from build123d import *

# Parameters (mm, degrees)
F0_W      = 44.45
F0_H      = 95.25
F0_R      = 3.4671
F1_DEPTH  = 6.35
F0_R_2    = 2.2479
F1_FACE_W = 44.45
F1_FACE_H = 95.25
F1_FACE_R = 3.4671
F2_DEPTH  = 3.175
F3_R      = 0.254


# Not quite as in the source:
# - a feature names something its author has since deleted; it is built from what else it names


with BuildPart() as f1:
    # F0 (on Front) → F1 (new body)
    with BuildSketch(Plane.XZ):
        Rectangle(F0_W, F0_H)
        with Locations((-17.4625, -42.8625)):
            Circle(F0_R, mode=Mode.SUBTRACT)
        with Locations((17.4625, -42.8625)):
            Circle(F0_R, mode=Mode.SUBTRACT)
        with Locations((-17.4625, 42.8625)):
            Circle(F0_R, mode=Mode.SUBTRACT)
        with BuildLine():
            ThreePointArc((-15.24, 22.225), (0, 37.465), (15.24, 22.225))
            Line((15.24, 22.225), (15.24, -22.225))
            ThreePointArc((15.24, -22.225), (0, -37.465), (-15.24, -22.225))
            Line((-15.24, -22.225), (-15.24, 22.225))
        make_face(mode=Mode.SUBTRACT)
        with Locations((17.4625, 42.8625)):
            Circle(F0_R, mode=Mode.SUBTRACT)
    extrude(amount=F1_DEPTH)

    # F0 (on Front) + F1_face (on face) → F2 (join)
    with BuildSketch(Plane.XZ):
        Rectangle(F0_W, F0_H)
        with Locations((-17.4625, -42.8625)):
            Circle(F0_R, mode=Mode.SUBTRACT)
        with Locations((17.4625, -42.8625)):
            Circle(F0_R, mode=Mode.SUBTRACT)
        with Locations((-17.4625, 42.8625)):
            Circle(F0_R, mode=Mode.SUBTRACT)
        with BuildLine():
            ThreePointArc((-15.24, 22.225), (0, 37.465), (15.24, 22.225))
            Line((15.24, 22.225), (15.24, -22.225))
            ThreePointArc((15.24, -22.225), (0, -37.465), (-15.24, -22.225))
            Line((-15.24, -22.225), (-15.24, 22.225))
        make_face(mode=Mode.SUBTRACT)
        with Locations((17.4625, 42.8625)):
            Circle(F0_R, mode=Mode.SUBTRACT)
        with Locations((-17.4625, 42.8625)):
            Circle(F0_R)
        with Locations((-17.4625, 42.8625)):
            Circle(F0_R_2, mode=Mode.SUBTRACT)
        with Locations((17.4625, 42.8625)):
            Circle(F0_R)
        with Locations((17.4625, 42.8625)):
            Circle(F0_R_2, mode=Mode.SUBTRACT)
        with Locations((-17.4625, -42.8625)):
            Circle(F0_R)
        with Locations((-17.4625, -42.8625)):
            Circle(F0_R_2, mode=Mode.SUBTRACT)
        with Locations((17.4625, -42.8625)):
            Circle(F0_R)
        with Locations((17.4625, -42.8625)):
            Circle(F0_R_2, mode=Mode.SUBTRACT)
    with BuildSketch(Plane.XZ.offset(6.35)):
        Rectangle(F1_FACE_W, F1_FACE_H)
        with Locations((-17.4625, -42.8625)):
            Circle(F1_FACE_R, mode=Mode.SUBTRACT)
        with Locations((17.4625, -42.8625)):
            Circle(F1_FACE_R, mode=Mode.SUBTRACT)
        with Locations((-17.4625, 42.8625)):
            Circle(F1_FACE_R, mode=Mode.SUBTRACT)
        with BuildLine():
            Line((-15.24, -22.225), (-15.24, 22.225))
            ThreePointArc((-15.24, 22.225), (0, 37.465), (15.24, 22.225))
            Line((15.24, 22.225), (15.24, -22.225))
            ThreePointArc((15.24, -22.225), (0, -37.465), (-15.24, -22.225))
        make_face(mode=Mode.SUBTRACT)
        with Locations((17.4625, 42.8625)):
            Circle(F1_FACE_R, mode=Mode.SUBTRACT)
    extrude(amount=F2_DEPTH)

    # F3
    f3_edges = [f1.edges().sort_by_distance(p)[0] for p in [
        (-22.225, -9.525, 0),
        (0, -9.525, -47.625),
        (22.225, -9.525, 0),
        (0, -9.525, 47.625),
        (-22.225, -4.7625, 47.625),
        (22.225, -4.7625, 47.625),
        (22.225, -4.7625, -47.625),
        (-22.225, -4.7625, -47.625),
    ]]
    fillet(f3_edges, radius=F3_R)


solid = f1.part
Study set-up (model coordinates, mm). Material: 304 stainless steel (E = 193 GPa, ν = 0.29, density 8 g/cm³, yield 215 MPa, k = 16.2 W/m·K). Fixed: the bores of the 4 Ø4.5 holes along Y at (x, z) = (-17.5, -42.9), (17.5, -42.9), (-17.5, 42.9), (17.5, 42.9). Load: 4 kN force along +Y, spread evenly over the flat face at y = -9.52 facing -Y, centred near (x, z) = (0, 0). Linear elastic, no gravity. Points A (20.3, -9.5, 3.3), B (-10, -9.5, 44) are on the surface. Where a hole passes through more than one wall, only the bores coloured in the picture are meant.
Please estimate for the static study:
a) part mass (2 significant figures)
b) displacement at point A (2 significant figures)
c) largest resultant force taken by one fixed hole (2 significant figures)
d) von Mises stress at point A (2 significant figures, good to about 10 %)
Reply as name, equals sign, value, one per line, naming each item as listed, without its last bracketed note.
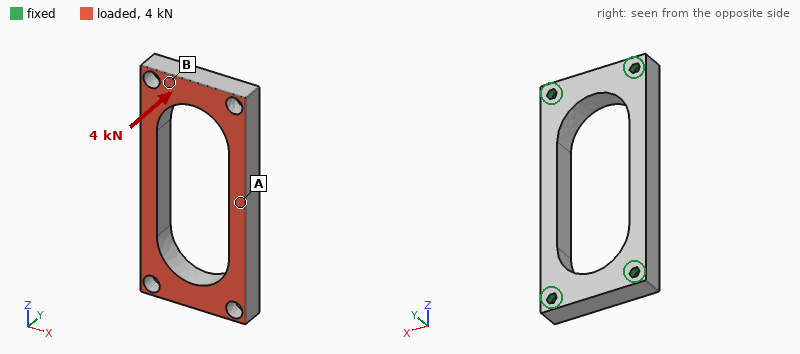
part mass = 150 g
displacement at point A = 32 µm
largest resultant force taken by one fixed hole = 1.3 kN
von Mises stress at point A = 58 MPa
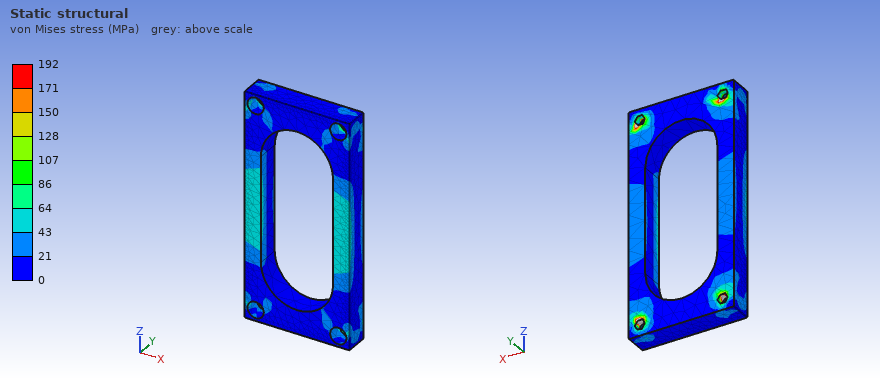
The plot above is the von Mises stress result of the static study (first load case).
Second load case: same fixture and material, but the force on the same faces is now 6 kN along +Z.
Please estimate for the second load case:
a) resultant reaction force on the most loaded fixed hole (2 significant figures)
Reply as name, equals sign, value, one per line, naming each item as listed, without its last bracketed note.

resultant reaction force on the most loaded fixed hole = 1.5 kN
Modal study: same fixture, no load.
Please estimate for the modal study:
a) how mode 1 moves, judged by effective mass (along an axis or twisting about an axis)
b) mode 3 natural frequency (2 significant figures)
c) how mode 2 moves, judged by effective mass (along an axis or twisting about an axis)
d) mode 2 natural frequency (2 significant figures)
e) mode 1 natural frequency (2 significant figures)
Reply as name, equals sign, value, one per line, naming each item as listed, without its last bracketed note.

how mode 1 moves, judged by effective mass = along Y
mode 3 natural frequency = 6300 Hz
how mode 2 moves, judged by effective mass = twisting about Z
mode 2 natural frequency = 5900 Hz
mode 1 natural frequency = 5200 Hz
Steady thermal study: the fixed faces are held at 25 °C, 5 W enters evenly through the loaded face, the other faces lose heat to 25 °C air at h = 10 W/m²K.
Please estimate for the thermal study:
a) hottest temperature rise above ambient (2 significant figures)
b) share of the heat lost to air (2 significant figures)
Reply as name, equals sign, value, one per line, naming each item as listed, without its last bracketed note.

hottest temperature rise above ambient = 14 K
share of the heat lost to air = 11 %
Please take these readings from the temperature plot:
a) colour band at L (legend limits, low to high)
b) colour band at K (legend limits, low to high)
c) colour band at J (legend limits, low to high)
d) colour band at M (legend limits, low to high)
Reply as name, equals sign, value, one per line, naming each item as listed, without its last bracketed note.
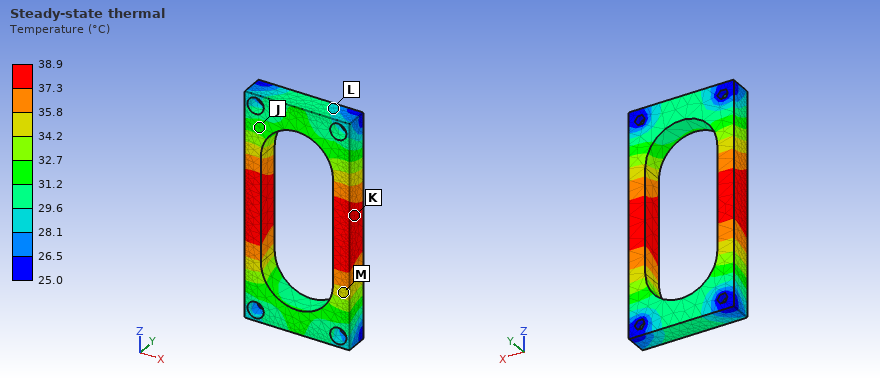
colour band at L = 28.1 to 29.6 °C
colour band at K = 37.3 to 38.9 °C
colour band at J = 31.2 to 32.7 °C
colour band at M = 34.2 to 35.8 °C
